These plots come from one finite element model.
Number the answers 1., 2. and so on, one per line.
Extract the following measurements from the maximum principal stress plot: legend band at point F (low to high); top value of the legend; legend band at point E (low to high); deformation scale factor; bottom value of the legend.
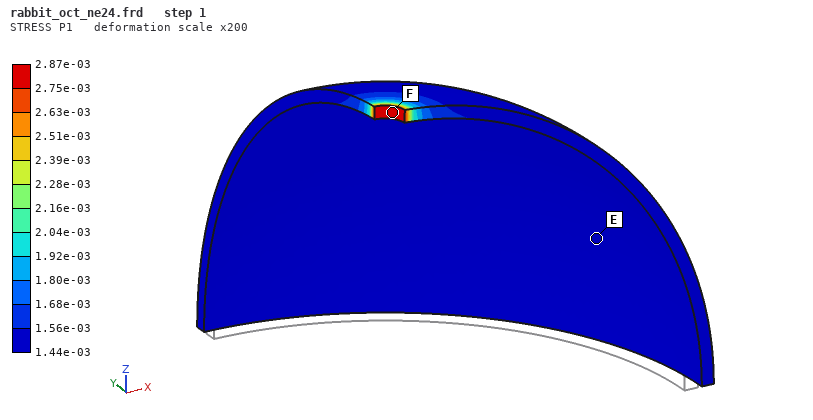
1. 2.75e-03 to 2.87e-03
2. 2.87e-03
3. 1.44e-03 to 1.56e-03
4. 200
5. 1.44e-03
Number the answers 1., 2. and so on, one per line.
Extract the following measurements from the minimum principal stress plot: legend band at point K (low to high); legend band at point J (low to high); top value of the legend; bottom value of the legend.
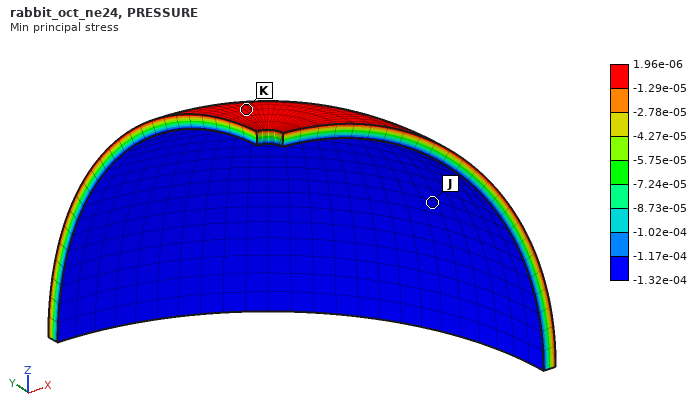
1. -1.29e-05 to 1.96e-06
2. -1.32e-04 to -1.17e-04
3. 1.96e-06
4. -1.32e-04
